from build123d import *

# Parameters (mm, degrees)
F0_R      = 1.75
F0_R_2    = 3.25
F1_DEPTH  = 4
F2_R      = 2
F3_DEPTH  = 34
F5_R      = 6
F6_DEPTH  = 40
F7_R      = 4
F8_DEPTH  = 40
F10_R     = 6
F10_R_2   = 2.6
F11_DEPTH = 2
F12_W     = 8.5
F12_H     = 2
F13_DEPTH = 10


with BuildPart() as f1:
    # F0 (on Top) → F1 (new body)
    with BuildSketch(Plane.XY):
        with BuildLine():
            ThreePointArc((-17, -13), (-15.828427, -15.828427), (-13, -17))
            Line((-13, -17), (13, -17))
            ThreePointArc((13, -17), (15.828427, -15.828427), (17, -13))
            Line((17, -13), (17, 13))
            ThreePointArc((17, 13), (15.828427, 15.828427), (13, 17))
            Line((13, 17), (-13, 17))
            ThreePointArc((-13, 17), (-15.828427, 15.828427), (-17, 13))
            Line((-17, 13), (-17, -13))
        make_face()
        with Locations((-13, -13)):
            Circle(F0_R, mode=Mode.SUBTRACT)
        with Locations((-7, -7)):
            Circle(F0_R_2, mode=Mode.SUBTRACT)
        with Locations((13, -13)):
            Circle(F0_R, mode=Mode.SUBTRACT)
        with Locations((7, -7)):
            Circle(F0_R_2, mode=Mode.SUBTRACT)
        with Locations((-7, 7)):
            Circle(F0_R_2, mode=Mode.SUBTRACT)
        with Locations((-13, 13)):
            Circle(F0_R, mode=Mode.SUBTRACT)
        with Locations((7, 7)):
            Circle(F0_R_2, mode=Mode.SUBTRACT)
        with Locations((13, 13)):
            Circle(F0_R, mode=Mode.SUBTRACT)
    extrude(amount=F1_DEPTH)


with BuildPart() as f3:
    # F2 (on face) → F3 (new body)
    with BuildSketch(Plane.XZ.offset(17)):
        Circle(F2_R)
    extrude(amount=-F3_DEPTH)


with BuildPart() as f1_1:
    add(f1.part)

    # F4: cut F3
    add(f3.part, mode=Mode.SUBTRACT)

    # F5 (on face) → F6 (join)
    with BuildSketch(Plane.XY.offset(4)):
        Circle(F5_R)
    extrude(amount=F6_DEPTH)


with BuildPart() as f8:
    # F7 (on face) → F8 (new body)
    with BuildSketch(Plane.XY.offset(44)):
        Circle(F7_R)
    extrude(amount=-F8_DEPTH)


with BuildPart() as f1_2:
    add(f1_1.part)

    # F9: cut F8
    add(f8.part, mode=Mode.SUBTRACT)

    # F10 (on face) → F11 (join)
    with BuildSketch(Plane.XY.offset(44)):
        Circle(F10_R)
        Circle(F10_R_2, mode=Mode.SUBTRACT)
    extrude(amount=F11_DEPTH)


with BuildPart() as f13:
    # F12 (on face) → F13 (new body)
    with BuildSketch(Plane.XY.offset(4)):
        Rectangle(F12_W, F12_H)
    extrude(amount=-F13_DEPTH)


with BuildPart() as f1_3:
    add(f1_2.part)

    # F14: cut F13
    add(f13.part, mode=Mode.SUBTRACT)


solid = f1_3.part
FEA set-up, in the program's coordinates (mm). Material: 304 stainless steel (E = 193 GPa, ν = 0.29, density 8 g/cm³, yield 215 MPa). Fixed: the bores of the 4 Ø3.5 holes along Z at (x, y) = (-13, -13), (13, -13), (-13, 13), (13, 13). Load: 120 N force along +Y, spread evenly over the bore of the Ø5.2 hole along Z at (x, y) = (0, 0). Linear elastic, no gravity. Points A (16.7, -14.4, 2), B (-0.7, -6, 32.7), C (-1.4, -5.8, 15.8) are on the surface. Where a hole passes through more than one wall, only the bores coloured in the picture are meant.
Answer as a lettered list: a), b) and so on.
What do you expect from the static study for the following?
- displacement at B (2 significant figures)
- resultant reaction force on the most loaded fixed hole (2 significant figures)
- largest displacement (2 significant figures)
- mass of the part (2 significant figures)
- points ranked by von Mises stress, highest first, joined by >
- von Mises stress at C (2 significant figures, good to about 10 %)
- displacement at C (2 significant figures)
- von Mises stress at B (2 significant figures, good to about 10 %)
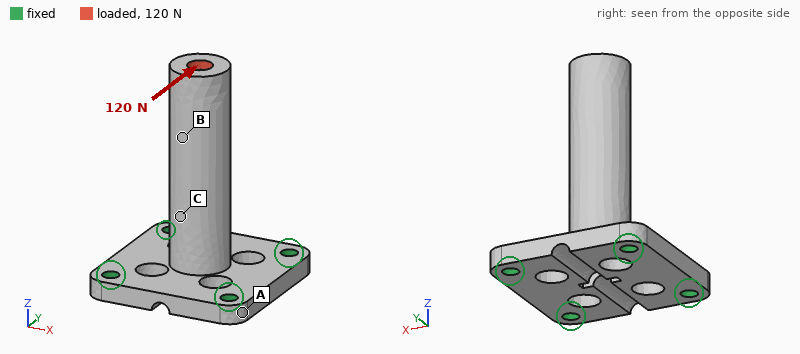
a) 32 µm
b) 160 N
c) 50 µm
d) 50 g
e) C > B > A
f) 25 MPa
g) 13 µm
h) 11 MPa
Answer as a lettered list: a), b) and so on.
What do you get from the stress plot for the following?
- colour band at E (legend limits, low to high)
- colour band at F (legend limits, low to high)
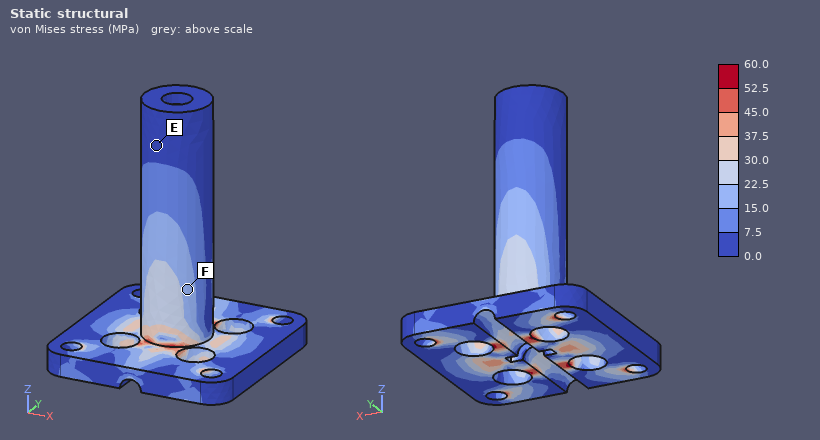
a) 0.0 to 7.5 MPa
b) 15.0 to 22.5 MPa
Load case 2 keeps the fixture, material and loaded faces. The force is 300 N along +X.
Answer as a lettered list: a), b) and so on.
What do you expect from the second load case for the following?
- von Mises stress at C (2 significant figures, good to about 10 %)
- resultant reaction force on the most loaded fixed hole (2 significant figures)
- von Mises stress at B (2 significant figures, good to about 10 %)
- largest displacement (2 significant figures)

a) 20 MPa
b) 310 N
c) 14 MPa
d) 0.11 mm
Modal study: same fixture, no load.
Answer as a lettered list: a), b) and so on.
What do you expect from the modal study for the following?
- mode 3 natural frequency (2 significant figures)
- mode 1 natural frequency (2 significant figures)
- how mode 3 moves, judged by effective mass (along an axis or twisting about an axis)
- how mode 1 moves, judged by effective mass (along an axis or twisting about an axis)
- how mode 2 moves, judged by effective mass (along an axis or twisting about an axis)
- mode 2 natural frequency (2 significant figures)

a) 9700 Hz
b) 2900 Hz
c) along Z
d) along Y
e) along X
f) 3100 Hz
